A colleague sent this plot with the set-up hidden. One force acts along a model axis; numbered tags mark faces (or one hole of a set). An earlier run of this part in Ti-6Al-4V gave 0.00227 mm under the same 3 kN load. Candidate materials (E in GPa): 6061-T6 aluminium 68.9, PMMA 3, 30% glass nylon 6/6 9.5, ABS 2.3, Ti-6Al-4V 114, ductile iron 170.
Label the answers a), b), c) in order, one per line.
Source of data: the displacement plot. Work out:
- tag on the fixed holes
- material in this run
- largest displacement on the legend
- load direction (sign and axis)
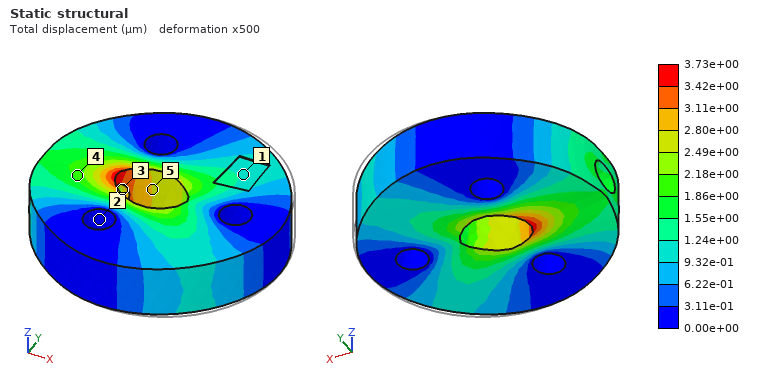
a) 2
b) 6061-T6 aluminium
c) 3.73e+00 µm
d) -X
